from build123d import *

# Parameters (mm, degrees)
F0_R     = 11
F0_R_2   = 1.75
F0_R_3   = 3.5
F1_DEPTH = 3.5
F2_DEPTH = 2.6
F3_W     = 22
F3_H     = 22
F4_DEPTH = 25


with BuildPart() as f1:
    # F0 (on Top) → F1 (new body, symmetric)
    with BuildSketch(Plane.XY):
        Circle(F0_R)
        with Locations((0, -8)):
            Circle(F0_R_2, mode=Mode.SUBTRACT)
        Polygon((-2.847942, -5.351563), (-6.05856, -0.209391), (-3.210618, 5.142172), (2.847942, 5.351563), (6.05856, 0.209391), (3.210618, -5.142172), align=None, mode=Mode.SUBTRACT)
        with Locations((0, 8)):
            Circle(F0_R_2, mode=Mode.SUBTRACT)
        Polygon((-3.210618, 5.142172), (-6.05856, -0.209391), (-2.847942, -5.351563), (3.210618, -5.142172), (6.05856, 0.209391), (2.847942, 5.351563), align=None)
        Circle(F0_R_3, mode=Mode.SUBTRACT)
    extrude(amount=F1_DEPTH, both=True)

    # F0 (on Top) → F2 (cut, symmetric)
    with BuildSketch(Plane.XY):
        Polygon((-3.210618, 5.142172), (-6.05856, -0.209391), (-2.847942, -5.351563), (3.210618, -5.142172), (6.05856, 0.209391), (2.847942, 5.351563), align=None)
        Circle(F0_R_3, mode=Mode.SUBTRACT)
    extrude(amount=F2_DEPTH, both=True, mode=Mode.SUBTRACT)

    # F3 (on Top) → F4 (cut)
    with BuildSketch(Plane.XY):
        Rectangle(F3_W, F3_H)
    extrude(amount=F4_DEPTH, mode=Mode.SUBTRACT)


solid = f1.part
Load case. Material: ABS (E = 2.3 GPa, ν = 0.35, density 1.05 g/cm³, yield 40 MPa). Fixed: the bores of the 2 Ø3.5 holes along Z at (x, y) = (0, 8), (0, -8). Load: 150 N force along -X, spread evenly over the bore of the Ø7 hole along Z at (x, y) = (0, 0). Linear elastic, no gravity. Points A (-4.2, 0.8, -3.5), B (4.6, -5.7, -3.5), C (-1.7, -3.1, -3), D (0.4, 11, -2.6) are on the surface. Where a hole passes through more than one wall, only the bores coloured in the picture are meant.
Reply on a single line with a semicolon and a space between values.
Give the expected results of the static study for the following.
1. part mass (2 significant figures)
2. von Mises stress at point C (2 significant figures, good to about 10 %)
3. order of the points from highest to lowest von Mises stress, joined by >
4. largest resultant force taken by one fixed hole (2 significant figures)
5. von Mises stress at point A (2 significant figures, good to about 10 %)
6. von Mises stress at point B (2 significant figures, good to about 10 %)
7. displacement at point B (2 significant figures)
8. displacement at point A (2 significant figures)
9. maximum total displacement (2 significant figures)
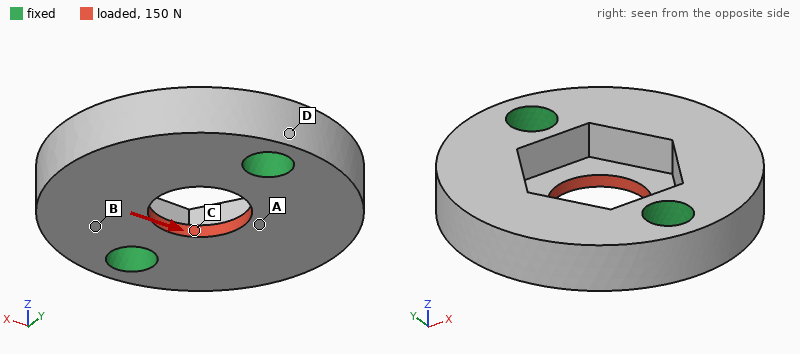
1.0 g; 13 MPa; C > A > B > D; 75 N; 7.4 MPa; 5.7 MPa; 12 µm; 29 µm; 40 µm
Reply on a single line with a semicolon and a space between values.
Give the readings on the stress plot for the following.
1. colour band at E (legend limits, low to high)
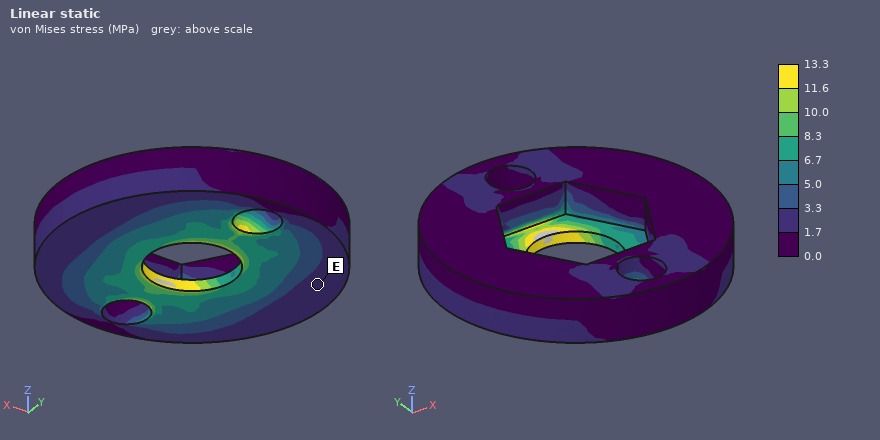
1.7 to 3.3 MPa
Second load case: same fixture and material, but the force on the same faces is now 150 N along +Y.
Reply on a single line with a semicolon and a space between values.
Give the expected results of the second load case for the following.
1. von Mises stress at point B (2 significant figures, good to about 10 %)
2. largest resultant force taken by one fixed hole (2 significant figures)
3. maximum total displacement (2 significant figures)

2.7 MPa; 75 N; 23 µm
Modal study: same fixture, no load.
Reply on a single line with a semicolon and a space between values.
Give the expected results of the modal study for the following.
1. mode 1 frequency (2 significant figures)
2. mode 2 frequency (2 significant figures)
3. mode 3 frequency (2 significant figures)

7000 Hz; 7300 Hz; 16 kHz
